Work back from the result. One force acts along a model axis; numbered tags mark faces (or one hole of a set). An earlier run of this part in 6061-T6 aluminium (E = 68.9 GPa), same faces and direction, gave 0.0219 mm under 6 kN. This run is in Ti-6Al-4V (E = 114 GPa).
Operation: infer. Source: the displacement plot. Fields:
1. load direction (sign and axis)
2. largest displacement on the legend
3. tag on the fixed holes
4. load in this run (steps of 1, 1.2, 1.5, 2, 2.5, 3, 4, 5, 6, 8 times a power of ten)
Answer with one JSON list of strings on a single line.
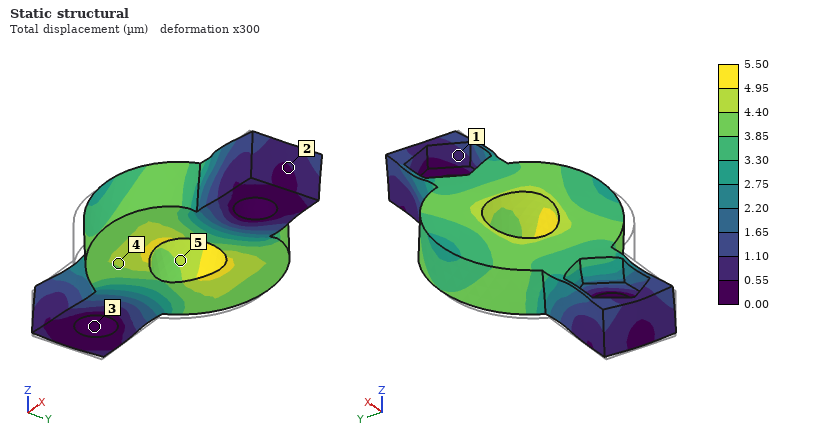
["+X", "5.50 µm", "3", "2.5 kN"]
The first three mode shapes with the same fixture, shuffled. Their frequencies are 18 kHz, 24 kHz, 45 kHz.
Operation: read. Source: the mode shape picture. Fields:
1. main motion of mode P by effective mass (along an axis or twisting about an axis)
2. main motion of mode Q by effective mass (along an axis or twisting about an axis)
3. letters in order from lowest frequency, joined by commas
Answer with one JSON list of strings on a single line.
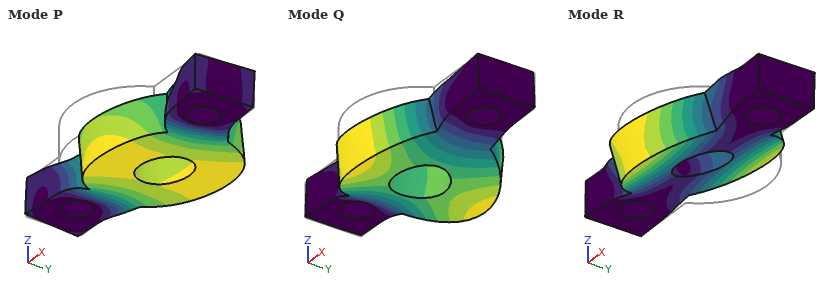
["along Y", "along Z", "R, Q, P"]
